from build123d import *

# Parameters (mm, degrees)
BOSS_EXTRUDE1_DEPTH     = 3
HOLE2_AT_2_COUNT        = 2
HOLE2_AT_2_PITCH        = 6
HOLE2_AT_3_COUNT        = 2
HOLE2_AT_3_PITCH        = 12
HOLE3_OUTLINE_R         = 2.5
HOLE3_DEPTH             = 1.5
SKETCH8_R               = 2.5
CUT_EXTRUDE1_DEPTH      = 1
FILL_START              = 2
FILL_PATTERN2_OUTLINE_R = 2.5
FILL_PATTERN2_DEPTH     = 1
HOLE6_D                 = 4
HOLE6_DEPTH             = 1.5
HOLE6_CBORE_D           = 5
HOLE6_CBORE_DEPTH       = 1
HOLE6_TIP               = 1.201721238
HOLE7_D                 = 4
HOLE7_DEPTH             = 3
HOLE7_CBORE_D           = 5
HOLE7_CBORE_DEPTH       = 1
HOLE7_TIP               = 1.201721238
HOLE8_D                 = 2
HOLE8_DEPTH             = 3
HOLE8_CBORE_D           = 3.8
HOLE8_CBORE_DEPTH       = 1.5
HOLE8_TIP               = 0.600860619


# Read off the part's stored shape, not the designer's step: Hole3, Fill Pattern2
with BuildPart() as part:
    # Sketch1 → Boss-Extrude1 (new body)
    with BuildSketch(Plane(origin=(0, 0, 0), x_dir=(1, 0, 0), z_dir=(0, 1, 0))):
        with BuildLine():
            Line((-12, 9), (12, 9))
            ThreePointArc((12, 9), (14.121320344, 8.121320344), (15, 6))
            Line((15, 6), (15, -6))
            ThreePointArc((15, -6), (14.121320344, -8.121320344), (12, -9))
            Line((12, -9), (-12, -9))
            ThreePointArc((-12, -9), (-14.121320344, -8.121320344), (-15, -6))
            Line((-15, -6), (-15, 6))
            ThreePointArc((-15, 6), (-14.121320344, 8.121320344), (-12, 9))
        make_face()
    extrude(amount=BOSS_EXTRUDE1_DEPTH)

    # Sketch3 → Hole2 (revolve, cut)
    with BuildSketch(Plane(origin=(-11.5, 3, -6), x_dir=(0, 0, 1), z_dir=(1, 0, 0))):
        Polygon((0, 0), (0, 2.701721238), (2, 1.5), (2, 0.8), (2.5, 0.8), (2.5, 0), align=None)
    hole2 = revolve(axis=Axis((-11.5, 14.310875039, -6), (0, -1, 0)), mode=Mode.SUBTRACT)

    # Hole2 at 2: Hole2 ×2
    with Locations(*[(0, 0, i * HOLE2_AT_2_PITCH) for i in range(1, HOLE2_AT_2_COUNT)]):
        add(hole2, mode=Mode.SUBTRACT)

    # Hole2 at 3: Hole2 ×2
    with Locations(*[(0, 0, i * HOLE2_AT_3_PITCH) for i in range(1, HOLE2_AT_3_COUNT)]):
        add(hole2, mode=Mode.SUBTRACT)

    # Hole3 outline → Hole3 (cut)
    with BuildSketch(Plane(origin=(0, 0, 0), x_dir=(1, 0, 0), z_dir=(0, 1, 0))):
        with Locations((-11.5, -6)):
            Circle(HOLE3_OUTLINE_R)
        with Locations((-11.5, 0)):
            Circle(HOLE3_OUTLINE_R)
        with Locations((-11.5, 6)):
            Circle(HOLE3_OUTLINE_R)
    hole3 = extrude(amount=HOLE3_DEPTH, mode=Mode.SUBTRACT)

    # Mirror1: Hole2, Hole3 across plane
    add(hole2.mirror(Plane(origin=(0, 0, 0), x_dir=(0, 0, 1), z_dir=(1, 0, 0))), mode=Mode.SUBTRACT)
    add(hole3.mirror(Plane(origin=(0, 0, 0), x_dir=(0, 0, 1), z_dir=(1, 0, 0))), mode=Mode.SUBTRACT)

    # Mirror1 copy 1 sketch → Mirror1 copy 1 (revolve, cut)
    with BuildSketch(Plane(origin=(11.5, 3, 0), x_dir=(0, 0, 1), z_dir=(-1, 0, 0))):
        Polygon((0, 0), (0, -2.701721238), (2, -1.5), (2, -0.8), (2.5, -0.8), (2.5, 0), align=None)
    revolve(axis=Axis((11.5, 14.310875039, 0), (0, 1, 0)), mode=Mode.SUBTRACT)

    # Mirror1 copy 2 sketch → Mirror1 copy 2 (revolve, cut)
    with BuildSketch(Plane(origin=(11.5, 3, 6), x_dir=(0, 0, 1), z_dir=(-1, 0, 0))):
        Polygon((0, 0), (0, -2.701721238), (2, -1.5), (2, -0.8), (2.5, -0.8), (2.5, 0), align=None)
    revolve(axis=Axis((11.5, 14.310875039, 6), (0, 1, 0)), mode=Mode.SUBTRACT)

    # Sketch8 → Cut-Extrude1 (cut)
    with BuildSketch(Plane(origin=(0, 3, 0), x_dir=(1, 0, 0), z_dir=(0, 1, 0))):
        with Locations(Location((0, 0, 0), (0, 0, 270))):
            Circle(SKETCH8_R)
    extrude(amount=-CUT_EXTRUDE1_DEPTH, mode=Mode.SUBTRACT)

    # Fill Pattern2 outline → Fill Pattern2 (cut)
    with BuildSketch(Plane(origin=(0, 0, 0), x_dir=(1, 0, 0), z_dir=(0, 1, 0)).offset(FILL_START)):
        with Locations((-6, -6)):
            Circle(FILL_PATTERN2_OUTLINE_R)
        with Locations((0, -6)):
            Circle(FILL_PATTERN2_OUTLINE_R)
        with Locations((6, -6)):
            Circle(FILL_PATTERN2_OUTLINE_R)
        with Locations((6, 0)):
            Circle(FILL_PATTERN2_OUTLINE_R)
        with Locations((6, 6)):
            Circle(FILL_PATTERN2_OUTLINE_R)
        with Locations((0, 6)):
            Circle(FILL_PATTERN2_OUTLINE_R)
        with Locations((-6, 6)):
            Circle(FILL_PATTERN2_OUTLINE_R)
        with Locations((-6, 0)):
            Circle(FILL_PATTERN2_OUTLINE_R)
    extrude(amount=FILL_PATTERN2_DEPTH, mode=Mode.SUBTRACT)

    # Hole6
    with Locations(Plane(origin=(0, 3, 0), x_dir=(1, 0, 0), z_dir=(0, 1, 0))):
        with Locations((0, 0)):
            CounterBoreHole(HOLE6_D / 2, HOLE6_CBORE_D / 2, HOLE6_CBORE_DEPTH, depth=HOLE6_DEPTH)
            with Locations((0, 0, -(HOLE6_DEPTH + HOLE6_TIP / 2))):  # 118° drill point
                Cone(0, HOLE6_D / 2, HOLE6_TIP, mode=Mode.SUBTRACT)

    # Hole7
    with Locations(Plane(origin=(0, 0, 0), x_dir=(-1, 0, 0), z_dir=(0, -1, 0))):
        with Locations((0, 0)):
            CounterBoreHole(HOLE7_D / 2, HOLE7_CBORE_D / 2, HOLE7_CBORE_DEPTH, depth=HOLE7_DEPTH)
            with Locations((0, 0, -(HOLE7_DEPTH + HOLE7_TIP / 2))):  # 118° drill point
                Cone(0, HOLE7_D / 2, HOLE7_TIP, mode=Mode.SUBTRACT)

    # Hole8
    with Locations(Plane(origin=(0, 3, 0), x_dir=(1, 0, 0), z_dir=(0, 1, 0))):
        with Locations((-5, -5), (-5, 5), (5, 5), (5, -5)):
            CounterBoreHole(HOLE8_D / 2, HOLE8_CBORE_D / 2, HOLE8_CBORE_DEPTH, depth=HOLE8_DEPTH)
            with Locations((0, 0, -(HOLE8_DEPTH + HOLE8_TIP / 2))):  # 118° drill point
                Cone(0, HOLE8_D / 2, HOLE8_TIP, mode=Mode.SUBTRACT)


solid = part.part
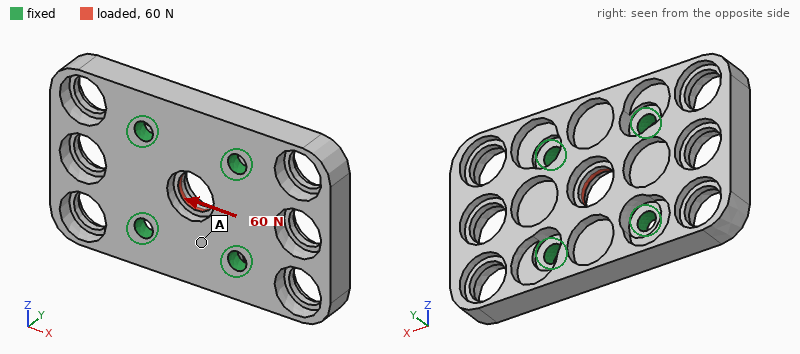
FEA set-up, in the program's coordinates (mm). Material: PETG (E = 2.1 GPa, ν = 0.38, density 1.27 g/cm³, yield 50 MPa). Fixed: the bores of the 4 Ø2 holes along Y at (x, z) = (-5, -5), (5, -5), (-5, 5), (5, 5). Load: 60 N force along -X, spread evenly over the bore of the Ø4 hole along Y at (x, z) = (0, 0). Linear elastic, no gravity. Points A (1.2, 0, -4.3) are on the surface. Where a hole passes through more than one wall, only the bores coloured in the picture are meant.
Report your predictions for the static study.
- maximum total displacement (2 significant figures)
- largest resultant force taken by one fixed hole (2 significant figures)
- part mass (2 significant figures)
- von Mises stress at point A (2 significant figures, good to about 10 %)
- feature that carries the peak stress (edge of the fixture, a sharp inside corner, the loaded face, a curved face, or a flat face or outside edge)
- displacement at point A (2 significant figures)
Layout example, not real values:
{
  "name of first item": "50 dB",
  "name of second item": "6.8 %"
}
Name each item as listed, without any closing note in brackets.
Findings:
{
  "maximum total displacement": "9.2 µm",
  "largest resultant force taken by one fixed hole": "16 N",
  "part mass": "1.3 g",
  "von Mises stress at point A": "1.2 MPa",
  "feature that carries the peak stress": "a sharp inside corner",
  "displacement at point A": "1.9 µm"
}
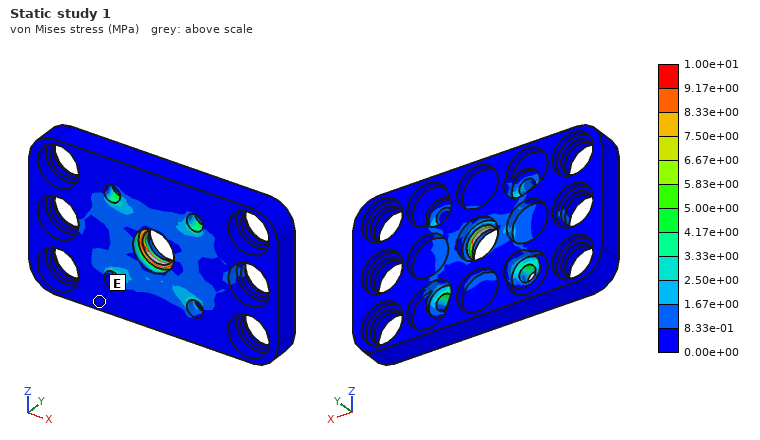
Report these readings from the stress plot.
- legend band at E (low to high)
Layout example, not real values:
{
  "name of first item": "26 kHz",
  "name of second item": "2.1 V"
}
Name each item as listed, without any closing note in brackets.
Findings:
{
  "legend band at E": "0.00e+00 to 8.33e-01 MPa"
}
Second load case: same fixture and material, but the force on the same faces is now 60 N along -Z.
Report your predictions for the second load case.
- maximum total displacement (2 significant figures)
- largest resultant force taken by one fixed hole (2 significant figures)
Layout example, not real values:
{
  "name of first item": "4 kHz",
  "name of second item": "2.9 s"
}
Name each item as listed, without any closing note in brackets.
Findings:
{
  "maximum total displacement": "9.3 µm",
  "largest resultant force taken by one fixed hole": "16 N"
}
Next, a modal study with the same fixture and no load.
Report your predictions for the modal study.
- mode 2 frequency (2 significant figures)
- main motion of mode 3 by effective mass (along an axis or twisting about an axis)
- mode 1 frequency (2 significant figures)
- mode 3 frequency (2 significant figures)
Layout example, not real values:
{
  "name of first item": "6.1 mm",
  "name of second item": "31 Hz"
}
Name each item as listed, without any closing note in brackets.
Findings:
{
  "mode 2 frequency": "4500 Hz",
  "main motion of mode 3 by effective mass": "twisting about X",
  "mode 1 frequency": "4400 Hz",
  "mode 3 frequency": "6700 Hz"
}
